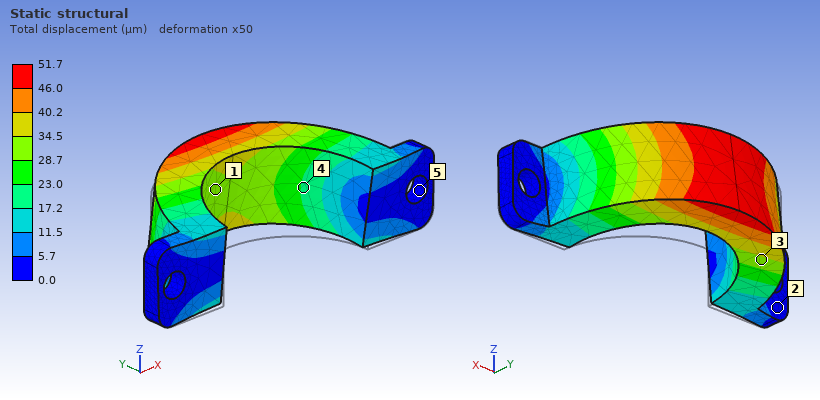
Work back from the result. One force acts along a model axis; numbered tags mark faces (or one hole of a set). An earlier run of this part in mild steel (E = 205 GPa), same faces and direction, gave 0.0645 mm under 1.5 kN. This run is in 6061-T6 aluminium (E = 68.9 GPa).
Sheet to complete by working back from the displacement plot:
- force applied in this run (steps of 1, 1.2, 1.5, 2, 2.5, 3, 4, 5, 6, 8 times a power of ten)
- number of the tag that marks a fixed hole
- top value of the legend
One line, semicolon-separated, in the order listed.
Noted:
400 N; 5; 51.7 µm
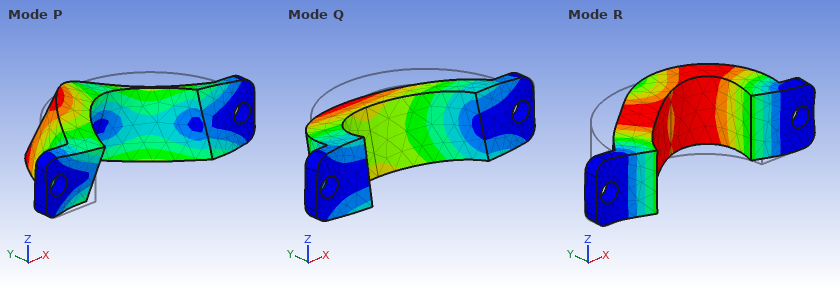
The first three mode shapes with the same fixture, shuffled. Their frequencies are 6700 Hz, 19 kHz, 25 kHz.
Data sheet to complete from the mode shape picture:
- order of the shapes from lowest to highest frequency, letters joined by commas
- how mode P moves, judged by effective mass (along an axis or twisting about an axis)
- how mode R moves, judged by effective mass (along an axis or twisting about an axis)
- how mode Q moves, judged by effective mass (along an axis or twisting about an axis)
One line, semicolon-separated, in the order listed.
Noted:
Q, R, P; twisting about Y; along X; along Z
